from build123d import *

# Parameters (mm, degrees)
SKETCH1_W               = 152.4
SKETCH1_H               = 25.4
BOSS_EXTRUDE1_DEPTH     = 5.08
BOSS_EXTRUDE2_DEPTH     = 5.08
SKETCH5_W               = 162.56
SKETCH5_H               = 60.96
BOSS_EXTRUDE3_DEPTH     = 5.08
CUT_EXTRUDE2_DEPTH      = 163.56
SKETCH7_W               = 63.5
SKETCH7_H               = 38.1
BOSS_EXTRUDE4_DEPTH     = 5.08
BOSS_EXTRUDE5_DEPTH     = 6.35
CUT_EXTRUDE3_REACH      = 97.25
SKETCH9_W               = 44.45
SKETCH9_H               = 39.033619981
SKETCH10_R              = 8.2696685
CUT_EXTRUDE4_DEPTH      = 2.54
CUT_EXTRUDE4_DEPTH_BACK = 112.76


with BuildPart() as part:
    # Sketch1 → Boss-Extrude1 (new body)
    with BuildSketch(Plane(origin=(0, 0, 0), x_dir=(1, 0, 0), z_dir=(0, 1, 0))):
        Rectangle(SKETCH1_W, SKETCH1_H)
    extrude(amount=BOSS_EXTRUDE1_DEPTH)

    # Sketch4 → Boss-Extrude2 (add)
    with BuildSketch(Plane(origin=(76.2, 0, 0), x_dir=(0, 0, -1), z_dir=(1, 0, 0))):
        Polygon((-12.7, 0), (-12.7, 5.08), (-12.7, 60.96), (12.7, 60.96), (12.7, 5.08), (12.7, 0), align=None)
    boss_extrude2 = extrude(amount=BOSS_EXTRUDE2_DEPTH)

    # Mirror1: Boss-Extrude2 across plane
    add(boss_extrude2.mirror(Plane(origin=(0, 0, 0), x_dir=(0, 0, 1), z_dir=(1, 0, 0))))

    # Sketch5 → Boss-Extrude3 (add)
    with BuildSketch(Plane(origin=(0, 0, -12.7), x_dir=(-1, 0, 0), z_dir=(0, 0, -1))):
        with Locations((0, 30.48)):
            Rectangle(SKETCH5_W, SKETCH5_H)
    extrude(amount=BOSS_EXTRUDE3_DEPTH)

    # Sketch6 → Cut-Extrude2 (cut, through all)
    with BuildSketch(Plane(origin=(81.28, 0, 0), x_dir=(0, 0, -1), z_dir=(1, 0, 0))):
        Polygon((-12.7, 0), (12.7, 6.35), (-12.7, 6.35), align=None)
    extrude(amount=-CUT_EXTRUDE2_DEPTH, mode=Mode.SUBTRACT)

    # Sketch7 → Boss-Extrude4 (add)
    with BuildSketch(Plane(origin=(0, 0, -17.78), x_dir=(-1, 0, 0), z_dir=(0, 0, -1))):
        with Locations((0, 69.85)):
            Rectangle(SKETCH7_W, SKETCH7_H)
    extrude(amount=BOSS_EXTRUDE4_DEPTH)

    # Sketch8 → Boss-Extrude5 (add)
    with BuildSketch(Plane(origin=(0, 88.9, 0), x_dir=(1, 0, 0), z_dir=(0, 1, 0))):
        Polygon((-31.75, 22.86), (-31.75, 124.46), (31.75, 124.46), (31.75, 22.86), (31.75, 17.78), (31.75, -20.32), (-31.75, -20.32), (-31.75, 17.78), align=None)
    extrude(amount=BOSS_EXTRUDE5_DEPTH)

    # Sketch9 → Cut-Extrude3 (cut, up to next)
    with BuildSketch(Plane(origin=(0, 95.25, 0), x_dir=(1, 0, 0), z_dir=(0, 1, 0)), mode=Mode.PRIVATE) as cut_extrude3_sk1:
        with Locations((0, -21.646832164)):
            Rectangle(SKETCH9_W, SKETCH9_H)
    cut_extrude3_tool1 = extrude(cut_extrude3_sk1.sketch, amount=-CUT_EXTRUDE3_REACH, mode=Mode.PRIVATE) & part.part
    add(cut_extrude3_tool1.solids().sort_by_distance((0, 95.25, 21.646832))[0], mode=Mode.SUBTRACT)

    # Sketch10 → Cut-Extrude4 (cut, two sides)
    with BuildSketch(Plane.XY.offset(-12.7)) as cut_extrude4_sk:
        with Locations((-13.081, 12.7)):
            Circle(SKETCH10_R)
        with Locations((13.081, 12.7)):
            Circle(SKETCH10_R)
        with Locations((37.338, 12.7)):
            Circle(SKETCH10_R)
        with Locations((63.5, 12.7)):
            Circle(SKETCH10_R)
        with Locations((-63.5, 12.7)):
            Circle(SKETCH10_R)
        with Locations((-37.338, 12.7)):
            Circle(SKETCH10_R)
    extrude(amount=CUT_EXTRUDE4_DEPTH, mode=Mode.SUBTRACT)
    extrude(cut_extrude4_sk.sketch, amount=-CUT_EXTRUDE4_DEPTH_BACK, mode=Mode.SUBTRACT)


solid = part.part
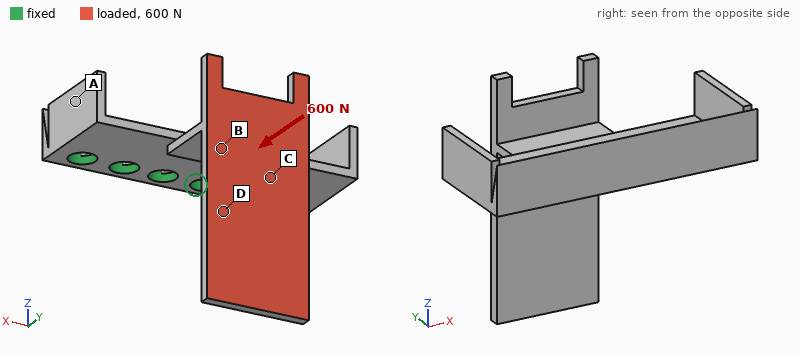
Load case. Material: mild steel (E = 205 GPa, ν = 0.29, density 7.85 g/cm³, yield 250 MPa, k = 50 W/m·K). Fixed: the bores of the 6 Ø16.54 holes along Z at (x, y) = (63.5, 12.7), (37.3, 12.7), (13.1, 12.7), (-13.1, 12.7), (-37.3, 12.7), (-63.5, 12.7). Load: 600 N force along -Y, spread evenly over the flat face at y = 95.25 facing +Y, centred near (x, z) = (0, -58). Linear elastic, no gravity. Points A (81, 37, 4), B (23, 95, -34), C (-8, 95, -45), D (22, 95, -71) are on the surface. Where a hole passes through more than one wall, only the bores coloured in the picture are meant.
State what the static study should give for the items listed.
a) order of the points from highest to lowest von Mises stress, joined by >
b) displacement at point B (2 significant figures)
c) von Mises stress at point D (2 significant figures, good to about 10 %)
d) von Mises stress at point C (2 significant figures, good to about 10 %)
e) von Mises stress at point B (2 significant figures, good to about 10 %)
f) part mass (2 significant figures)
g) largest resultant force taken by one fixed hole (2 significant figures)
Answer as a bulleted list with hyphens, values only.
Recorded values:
- B > C > D > A
- 0.30 mm
- 15 MPa
- 31 MPa
- 41 MPa
- 1.1 kg
- 340 N
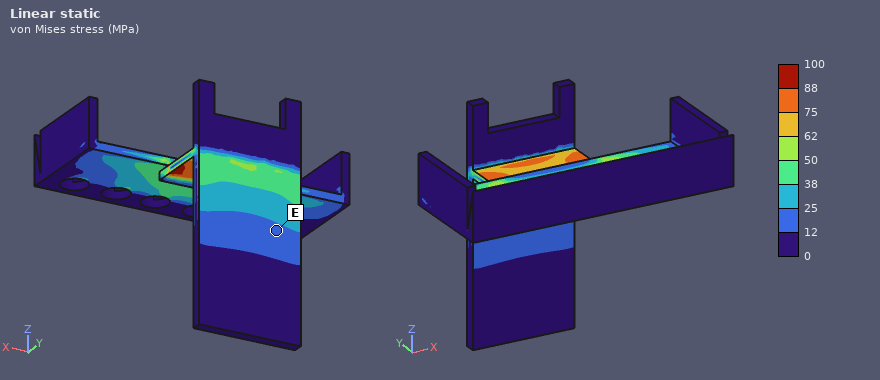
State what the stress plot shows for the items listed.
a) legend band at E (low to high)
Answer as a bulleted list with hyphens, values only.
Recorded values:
- 12 to 25 MPa
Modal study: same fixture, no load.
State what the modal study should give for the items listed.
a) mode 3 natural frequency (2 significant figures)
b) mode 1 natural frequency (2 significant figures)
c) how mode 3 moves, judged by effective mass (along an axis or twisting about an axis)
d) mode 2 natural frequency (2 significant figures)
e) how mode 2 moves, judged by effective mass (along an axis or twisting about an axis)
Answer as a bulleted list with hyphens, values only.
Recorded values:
- 610 Hz
- 200 Hz
- along Z
- 420 Hz
- along X
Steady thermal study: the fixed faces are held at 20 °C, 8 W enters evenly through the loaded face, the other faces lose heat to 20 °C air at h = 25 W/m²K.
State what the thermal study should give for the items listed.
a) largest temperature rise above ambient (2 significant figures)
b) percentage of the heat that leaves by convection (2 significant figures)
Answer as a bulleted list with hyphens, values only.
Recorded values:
- 18 K
- 67 %
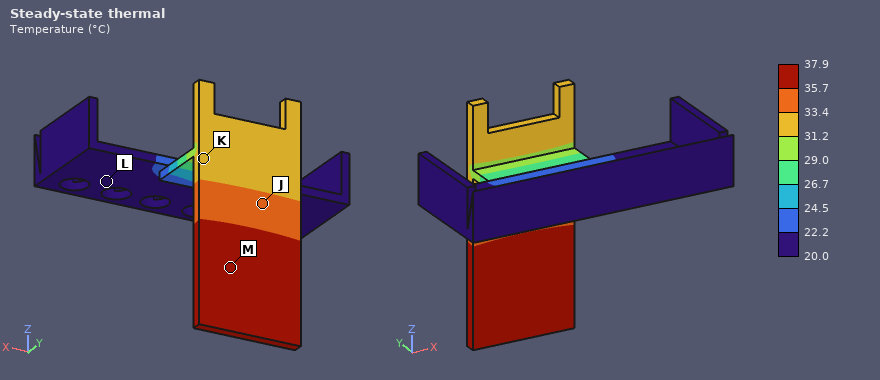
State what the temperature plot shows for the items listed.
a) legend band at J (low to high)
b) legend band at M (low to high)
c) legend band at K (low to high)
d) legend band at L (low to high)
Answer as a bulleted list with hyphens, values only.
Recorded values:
- 33.4 to 35.7 °C
- 35.7 to 37.9 °C
- 31.2 to 33.4 °C
- 20.0 to 22.2 °C
